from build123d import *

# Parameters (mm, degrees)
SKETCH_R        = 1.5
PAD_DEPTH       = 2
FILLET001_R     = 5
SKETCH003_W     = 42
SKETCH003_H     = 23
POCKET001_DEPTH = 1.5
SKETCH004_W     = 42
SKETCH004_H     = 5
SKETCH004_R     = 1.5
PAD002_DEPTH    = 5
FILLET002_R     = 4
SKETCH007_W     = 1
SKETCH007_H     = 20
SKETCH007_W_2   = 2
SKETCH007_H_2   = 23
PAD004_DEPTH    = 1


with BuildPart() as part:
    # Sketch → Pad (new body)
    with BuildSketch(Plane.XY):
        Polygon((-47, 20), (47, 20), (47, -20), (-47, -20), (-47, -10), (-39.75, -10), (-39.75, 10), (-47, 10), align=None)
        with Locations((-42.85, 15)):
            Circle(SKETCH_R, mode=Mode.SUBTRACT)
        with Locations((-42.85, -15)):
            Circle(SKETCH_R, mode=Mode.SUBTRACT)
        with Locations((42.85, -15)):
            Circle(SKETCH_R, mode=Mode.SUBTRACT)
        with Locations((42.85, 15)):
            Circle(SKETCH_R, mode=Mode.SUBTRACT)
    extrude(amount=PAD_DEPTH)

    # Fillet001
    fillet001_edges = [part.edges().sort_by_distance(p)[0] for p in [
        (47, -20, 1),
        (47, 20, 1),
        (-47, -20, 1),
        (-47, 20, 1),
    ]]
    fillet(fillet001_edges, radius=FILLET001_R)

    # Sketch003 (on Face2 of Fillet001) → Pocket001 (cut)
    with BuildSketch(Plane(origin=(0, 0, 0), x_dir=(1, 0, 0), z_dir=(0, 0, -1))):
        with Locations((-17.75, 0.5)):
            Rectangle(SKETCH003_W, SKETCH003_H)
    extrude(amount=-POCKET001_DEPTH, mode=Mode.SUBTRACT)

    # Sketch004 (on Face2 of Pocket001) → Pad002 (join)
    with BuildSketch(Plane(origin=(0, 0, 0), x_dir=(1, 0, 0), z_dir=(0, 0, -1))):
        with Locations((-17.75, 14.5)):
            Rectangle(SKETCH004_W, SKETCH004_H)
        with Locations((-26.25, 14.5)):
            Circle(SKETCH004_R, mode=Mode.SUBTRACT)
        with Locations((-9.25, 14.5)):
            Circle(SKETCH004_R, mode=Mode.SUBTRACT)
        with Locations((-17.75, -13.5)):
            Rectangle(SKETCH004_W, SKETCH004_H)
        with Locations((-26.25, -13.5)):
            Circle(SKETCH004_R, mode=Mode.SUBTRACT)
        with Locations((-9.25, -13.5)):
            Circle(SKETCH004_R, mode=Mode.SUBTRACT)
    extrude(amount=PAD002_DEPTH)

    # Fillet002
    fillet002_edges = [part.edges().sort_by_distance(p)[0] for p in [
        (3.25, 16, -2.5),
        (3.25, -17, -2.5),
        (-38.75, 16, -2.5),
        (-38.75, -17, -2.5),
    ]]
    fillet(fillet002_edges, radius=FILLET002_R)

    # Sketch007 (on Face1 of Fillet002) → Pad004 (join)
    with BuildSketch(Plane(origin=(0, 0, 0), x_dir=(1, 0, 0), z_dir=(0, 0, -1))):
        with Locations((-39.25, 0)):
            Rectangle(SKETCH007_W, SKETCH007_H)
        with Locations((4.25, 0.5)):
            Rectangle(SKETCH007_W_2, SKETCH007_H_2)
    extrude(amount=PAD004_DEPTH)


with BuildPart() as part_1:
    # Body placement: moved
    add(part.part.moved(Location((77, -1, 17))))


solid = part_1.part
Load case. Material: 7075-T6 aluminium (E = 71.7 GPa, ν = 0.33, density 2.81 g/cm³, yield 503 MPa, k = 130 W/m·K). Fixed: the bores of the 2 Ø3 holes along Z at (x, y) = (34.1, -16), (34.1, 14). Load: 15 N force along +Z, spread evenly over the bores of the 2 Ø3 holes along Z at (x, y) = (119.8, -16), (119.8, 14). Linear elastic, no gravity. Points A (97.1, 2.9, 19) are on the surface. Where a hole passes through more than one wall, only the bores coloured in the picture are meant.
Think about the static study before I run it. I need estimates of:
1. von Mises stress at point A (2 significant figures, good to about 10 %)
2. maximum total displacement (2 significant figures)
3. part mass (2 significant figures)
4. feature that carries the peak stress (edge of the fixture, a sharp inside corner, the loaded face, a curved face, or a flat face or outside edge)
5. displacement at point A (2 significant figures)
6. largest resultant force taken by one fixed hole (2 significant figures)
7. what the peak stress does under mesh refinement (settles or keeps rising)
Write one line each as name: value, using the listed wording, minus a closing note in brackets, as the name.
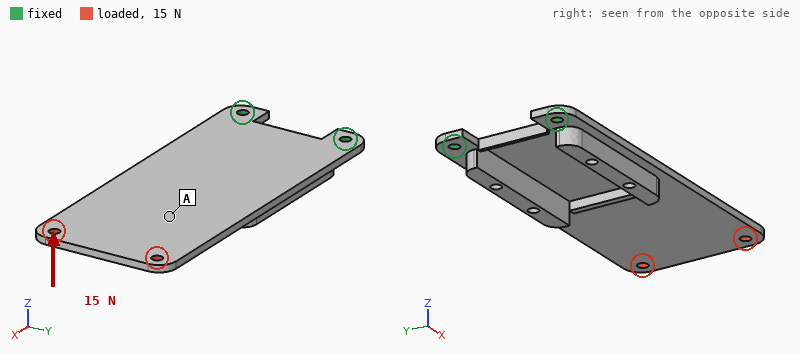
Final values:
von Mises stress at point A: 13 MPa
maximum total displacement: 0.94 mm
part mass: 21 g
feature that carries the peak stress: edge of the fixture
displacement at point A: 0.53 mm
largest resultant force taken by one fixed hole: 11 N
what the peak stress does under mesh refinement: keeps rising
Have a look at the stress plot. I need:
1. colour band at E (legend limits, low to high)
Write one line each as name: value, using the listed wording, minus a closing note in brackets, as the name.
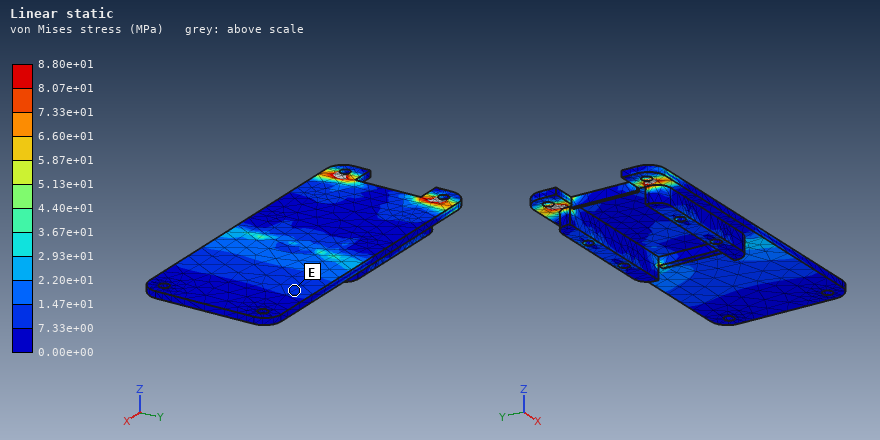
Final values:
colour band at E: 7.33e+00 to 1.47e+01 MPa
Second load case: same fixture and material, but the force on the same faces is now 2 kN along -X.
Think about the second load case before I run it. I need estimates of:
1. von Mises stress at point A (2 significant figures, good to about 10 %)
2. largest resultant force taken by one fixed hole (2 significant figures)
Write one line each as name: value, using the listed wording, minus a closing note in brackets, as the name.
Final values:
von Mises stress at point A: 17 MPa
largest resultant force taken by one fixed hole: 1.0 kN
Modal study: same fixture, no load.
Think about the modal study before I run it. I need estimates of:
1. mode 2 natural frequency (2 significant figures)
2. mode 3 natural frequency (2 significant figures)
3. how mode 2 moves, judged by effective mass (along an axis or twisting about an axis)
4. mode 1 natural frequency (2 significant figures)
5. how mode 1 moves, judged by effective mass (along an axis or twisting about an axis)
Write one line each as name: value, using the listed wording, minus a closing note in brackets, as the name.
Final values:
mode 2 natural frequency: 1100 Hz
mode 3 natural frequency: 1400 Hz
how mode 2 moves, judged by effective mass: twisting about X
mode 1 natural frequency: 270 Hz
how mode 1 moves, judged by effective mass: along Z
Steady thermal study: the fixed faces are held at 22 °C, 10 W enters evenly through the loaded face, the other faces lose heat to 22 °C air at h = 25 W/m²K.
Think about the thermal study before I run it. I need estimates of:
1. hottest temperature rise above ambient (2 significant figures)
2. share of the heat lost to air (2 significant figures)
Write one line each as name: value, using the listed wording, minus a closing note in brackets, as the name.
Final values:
hottest temperature rise above ambient: 62 K
share of the heat lost to air: 55 %
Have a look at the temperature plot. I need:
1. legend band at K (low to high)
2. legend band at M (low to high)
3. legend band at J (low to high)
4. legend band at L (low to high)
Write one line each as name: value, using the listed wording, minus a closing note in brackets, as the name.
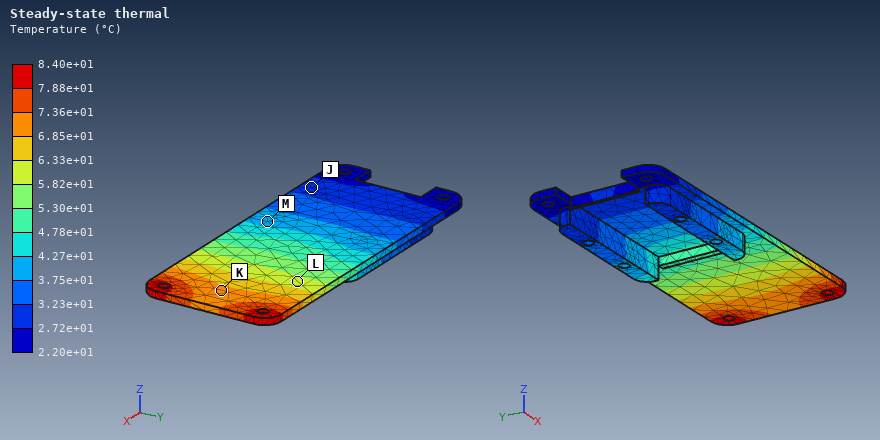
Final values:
legend band at K: 6.85e+01 to 7.36e+01 °C
legend band at M: 3.75e+01 to 4.27e+01 °C
legend band at J: 2.72e+01 to 3.23e+01 °C
legend band at L: 5.82e+01 to 6.33e+01 °C
